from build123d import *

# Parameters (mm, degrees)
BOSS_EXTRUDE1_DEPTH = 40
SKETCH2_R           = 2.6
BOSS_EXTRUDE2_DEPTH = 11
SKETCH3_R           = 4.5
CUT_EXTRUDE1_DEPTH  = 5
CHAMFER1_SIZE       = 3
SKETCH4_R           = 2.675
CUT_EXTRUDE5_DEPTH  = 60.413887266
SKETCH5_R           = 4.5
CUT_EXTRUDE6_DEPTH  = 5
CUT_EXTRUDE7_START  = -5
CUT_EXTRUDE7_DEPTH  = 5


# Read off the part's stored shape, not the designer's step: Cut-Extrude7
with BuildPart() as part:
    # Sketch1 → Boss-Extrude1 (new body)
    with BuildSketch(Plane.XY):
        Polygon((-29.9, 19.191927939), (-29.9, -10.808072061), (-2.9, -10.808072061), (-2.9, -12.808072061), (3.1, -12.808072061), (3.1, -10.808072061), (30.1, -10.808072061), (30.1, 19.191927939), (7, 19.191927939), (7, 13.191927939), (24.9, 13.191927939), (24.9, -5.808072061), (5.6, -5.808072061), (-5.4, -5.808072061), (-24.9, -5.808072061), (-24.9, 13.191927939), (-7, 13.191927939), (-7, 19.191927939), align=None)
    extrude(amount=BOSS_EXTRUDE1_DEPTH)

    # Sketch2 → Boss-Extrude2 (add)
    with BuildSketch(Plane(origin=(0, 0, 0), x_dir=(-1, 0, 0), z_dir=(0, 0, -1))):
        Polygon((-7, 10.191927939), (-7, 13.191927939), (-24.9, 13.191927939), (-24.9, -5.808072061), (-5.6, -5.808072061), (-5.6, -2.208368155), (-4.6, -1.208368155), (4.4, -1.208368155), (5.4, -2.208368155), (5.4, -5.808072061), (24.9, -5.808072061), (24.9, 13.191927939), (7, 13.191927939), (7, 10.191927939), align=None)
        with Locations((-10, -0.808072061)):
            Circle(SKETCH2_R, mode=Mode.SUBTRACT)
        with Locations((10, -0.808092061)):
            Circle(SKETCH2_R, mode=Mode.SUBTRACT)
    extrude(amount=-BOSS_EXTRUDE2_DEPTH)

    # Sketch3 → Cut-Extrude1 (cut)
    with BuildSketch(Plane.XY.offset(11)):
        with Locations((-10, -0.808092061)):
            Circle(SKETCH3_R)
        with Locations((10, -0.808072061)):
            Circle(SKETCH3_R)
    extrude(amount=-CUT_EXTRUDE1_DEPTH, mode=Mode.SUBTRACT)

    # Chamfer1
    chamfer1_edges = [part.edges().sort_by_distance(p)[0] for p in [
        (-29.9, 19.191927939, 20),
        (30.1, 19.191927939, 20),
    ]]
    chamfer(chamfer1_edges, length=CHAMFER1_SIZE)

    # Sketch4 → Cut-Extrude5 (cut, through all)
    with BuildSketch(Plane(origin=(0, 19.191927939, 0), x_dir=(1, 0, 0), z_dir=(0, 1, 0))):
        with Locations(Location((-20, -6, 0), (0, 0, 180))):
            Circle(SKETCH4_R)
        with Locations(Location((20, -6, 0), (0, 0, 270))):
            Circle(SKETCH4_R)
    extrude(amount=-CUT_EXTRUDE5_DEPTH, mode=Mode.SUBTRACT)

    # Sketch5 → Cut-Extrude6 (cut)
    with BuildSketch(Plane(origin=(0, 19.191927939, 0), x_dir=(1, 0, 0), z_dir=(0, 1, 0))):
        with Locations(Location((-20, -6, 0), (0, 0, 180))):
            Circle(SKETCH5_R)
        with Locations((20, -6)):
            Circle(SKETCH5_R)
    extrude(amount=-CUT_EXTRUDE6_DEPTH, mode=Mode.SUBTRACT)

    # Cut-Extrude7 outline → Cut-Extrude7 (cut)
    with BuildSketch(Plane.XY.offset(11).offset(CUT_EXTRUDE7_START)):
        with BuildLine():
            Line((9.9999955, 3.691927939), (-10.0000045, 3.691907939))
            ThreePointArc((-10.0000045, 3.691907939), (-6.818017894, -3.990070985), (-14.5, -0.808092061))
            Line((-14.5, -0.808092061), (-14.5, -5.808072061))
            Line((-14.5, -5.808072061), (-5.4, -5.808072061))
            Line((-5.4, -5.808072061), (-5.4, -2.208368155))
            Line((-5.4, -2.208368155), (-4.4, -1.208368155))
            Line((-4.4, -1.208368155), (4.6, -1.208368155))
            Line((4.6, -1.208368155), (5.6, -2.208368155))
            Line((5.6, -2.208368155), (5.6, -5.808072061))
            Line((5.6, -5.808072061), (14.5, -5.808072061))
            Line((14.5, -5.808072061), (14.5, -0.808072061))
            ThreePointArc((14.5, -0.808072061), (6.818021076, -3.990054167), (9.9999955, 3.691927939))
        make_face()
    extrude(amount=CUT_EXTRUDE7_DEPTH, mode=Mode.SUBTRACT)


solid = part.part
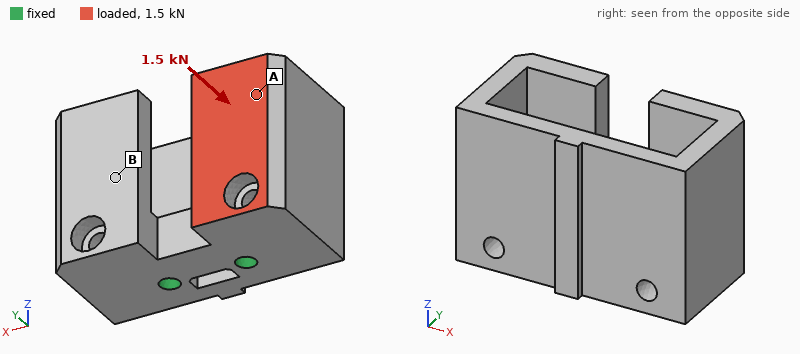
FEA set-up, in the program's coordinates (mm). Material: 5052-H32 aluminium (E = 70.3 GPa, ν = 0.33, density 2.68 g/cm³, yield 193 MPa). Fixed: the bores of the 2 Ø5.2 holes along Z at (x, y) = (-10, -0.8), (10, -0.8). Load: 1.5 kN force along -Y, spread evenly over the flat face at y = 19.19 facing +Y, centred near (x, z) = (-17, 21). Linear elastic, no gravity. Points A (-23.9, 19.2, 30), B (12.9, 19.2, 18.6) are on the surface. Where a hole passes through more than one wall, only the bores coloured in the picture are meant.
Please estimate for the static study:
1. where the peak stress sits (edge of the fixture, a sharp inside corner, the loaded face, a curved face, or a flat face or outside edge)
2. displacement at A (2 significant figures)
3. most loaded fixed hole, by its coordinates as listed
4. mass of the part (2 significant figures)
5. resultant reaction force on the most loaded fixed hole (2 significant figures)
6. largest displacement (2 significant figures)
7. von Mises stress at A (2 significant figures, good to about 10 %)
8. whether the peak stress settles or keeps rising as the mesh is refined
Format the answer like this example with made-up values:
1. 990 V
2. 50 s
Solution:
1. edge of the fixture
2. 0.11 mm
3. (-10, -0.8)
4. 100 g
5. 1.7 kN
6. 0.18 mm
7. 24 MPa
8. keeps rising
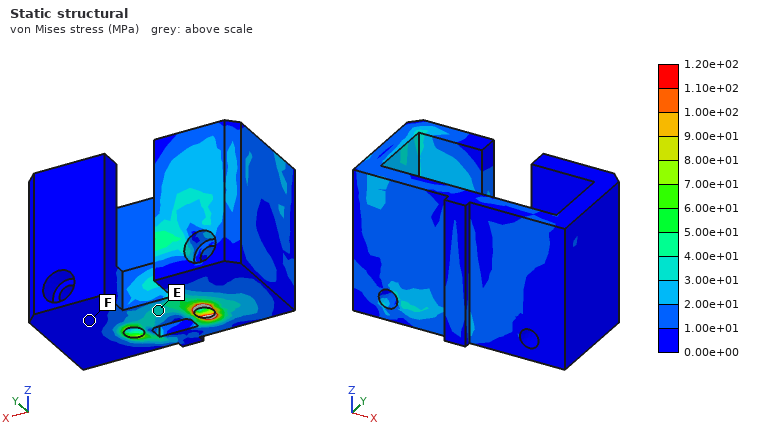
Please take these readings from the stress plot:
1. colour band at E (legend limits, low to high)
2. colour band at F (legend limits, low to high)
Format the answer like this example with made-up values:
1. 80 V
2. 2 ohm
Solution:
1. 3.00e+01 to 4.00e+01 MPa
2. 0.00e+00 to 1.00e+01 MPa
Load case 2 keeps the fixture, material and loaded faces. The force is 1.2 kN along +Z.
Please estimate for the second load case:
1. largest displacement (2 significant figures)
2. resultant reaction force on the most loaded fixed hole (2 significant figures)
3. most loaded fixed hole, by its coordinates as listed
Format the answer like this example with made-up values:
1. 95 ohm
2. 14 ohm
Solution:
1. 0.12 mm
2. 1.4 kN
3. (-10, -0.8)
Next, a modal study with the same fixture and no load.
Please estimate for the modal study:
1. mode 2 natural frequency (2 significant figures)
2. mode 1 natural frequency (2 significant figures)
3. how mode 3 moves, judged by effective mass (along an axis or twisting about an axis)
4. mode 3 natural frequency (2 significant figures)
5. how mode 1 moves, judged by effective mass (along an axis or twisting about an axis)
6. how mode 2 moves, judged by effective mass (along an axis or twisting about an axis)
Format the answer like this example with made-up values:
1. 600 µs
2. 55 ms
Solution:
1. 3900 Hz
2. 2800 Hz
3. along X
4. 4600 Hz
5. along Y
6. twisting about Z
